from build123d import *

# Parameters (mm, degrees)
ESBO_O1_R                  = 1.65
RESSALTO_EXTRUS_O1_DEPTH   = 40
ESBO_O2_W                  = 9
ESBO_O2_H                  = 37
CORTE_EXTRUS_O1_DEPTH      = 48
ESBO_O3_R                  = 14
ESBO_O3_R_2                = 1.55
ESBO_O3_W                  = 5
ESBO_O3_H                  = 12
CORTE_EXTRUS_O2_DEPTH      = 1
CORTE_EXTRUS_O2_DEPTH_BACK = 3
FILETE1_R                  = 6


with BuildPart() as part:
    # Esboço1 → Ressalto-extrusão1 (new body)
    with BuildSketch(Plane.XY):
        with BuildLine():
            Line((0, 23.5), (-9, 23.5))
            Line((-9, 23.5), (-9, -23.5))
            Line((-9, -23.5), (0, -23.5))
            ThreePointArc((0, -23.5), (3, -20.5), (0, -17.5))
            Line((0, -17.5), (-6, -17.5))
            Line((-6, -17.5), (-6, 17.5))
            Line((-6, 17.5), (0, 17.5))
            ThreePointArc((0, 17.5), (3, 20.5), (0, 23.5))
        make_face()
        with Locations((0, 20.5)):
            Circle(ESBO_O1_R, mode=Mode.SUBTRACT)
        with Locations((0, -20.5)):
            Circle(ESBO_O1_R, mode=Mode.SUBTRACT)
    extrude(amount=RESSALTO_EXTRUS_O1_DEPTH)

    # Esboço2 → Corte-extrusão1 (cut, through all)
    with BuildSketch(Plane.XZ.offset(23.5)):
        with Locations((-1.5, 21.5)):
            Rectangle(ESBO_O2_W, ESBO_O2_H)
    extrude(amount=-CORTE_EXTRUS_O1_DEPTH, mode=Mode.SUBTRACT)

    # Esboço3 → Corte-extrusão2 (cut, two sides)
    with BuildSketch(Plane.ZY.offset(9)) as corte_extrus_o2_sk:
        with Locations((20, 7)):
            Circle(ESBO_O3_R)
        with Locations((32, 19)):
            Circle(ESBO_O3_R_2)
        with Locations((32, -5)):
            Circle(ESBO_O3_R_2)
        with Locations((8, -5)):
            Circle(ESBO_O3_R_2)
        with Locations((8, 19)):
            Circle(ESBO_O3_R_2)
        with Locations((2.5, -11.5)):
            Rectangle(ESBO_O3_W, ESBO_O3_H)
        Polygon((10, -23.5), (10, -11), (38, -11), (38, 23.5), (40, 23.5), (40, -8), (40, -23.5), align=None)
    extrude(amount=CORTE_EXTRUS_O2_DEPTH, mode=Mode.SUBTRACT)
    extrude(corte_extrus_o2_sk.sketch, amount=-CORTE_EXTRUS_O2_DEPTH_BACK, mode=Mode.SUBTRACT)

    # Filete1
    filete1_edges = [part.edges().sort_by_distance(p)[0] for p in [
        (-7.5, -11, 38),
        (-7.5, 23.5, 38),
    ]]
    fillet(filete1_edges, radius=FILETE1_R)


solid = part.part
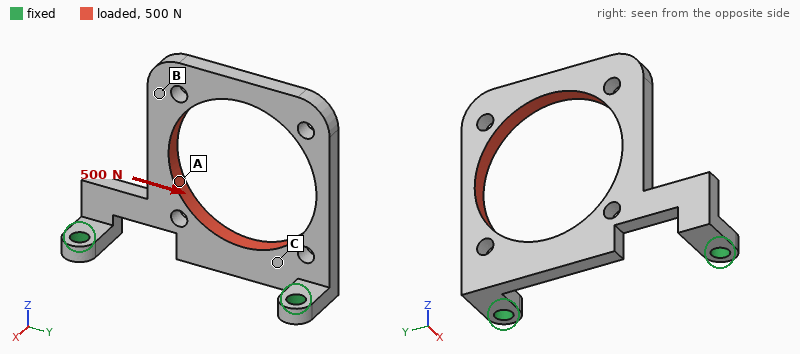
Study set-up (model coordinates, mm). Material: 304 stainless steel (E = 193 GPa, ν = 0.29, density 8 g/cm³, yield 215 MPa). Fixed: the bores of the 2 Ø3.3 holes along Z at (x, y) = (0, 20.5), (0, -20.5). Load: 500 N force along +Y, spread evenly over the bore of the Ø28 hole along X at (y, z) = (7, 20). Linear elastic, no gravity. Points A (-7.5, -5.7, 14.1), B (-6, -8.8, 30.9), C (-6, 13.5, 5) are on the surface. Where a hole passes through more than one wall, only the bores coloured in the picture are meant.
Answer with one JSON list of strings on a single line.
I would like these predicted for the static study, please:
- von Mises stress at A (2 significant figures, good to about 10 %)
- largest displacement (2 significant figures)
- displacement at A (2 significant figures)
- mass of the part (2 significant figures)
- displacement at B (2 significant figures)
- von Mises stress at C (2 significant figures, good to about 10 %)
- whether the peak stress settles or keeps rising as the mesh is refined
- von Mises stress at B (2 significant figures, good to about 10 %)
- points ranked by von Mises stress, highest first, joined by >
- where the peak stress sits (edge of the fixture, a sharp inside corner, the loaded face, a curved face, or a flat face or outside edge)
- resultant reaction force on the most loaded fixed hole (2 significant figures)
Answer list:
["100 MPa", "60 µm", "12 µm", "19 g", "48 µm", "27 MPa", "keeps rising", "12 MPa", "A > C > B", "edge of the fixture", "340 N"]
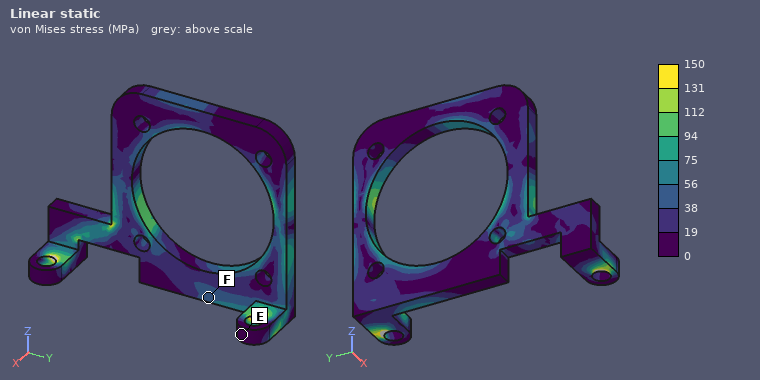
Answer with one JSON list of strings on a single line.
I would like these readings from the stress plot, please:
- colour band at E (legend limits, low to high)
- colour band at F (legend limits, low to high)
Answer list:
["0 to 19 MPa", "38 to 56 MPa"]
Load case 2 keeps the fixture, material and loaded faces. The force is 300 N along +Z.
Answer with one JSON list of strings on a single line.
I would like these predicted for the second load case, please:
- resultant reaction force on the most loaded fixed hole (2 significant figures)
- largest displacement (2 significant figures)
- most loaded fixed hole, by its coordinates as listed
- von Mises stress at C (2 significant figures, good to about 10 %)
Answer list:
["210 N", "51 µm", "(0, 20.5)", "9.9 MPa"]
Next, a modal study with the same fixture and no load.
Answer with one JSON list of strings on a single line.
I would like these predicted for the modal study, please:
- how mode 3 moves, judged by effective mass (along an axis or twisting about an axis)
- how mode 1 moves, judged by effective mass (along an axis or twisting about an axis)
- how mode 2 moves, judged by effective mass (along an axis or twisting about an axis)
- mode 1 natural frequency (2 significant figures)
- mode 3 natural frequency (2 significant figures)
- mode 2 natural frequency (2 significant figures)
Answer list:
["along Y", "along X", "twisting about Z", "1000 Hz", "4500 Hz", "2900 Hz"]
